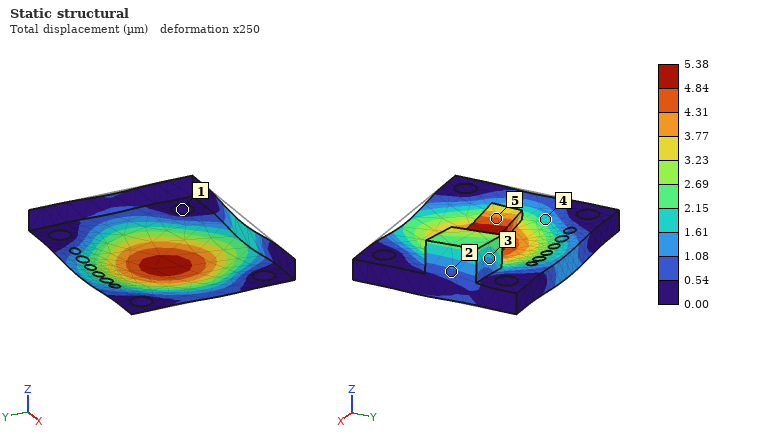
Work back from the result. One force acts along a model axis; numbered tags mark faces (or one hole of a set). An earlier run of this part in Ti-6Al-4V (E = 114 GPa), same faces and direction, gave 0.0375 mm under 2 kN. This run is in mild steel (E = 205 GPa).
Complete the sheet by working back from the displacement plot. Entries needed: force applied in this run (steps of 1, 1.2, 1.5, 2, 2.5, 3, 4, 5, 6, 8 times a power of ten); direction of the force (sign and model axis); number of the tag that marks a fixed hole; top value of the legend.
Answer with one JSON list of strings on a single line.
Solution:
["500 N", "-Z", "1", "5.38 µm"]
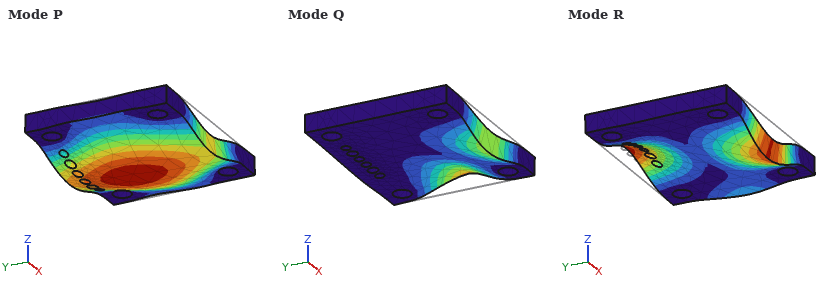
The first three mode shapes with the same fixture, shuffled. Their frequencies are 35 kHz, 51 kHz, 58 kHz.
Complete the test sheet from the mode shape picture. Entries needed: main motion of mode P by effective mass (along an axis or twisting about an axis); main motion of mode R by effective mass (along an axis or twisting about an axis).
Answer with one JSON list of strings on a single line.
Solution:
["along Z", "twisting about X"]
